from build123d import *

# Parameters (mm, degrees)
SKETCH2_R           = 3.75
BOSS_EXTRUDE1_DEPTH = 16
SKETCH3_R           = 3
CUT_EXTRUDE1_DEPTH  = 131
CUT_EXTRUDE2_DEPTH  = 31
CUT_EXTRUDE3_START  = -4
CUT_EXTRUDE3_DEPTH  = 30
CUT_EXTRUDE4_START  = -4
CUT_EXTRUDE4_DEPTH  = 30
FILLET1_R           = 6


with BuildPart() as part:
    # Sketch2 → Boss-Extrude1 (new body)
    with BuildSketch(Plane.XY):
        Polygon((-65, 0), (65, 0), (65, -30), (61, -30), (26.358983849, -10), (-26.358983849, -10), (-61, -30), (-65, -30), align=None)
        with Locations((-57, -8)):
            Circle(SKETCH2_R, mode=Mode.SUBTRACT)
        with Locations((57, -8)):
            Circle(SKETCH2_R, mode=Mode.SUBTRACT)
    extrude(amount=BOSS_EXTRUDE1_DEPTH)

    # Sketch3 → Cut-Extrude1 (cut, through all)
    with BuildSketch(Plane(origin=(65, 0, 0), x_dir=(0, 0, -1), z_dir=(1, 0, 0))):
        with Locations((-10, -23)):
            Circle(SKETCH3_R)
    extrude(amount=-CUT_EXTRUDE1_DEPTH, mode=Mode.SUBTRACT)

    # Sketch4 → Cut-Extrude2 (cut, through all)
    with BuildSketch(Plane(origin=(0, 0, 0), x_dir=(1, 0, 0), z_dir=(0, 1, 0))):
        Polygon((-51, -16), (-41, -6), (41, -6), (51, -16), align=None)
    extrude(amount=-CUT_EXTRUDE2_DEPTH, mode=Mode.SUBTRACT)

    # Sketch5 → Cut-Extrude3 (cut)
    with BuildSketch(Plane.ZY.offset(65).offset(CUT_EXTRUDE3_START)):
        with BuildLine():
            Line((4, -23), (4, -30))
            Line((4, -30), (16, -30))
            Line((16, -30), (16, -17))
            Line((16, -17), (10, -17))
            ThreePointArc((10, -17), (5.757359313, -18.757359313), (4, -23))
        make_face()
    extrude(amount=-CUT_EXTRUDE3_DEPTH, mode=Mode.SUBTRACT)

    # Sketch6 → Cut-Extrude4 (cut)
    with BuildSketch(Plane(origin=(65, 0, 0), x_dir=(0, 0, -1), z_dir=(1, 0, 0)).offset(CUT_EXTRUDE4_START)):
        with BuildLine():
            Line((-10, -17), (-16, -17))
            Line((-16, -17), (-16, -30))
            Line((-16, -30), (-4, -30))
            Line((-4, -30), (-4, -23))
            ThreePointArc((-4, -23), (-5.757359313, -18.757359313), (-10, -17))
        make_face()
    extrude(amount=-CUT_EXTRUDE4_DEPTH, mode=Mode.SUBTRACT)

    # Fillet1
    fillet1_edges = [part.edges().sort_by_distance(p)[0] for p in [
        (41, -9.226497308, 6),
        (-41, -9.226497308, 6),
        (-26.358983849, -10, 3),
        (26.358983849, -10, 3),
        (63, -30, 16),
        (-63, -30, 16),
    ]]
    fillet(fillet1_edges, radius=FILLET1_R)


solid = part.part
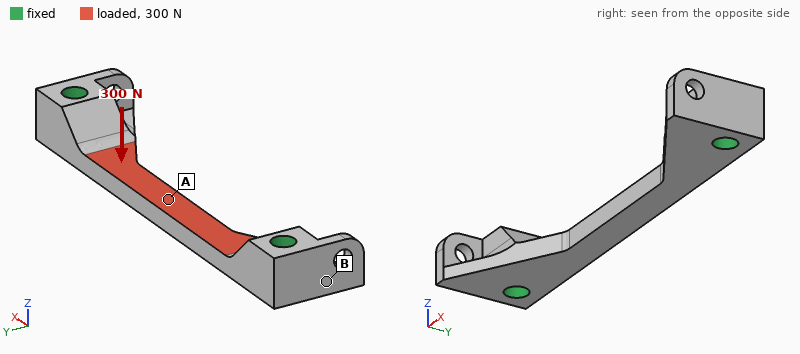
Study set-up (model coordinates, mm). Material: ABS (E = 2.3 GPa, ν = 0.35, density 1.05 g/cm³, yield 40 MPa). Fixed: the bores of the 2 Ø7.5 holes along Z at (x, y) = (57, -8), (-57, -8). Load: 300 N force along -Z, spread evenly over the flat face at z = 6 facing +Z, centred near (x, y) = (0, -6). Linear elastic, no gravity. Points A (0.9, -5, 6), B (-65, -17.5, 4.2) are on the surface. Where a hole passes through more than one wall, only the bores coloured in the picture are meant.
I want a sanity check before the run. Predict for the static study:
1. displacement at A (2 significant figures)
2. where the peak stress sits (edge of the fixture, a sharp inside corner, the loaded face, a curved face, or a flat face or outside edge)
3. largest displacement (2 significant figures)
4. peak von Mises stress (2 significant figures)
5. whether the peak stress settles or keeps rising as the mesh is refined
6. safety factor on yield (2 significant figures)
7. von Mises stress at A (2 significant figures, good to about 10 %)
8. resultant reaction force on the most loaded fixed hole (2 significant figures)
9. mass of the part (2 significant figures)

1.2 mm
a curved face
1.3 mm
24 MPa
settles
1.7
16 MPa
160 N
19 g
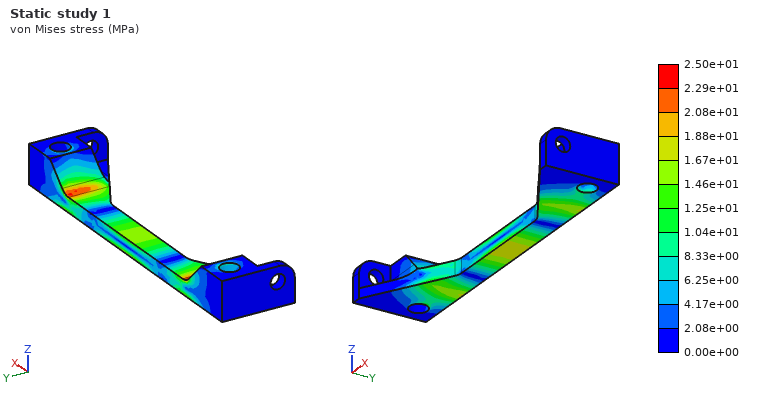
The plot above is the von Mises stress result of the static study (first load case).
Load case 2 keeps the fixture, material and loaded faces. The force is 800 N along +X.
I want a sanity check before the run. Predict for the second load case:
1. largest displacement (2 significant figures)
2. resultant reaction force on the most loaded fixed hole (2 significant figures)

96 µm
400 N
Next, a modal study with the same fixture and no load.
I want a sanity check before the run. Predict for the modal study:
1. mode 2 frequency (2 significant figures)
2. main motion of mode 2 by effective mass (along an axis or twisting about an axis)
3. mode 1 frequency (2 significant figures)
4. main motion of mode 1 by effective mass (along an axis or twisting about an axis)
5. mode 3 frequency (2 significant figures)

2100 Hz
along Y
1200 Hz
along Z
3000 Hz
